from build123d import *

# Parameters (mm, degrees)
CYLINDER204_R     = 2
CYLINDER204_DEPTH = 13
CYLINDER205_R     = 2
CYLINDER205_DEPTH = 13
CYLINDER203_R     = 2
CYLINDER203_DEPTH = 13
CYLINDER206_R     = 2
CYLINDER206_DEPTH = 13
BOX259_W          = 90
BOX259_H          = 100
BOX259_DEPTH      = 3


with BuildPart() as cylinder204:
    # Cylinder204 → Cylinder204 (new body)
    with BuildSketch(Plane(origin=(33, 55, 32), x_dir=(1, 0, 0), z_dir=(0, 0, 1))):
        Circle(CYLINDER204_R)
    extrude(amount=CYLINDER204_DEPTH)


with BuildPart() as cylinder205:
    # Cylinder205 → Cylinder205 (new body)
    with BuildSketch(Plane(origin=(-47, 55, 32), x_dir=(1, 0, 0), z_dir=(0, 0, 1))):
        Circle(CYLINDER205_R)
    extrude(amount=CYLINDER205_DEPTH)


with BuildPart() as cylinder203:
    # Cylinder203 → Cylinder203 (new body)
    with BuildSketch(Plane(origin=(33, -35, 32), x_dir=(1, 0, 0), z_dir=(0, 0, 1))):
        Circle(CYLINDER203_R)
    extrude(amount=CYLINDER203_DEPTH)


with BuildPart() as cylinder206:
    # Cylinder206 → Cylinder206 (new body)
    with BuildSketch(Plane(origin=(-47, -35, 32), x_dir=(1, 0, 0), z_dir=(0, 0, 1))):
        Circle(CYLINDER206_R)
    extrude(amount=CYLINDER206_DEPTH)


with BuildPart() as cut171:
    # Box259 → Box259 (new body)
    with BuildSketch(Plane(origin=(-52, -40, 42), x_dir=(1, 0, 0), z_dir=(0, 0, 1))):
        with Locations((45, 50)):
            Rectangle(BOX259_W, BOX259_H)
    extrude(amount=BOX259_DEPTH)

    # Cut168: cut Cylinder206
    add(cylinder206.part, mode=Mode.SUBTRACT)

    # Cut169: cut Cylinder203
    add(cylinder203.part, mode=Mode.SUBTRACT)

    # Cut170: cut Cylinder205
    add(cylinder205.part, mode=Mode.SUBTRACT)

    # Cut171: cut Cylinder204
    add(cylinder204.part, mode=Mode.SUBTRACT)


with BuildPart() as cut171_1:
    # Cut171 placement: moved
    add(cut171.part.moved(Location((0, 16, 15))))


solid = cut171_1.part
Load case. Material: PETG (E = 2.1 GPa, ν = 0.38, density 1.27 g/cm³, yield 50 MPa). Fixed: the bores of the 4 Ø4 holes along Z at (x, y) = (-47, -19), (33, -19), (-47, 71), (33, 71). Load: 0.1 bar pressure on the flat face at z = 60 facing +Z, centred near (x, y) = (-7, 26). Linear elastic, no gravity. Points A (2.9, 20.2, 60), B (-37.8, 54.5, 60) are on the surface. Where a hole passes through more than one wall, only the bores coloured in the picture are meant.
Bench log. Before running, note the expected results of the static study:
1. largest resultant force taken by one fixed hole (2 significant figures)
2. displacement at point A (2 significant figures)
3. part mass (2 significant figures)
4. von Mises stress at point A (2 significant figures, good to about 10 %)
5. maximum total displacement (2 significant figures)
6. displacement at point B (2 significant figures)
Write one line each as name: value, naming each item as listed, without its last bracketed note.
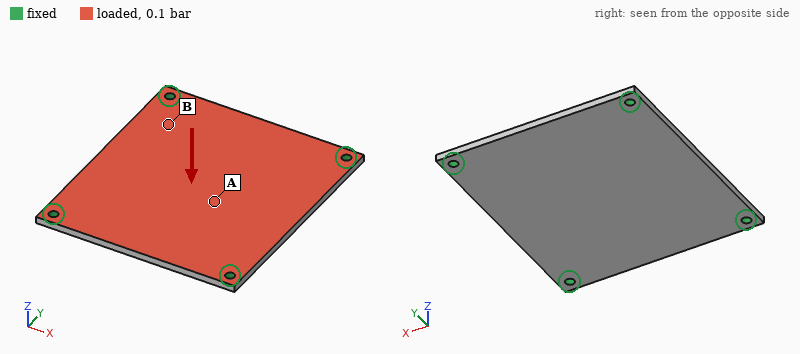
largest resultant force taken by one fixed hole: 22 N
displacement at point A: 0.77 mm
part mass: 34 g
von Mises stress at point A: 2.8 MPa
maximum total displacement: 0.80 mm
displacement at point B: 0.32 mm
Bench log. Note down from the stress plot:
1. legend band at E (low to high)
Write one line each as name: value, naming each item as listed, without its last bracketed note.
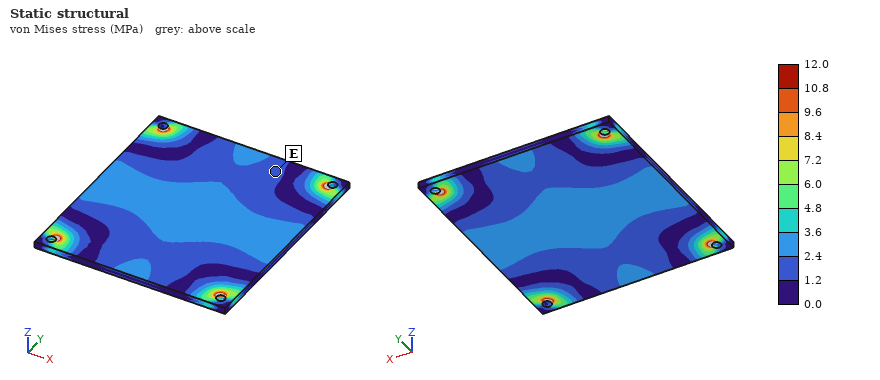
legend band at E: 1.2 to 2.4 MPa
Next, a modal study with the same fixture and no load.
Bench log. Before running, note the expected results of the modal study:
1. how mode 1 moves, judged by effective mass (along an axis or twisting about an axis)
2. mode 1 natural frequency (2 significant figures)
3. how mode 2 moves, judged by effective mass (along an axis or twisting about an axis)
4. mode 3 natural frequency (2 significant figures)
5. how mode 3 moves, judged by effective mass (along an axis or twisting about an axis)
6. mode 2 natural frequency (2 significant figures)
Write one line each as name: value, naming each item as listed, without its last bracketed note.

how mode 1 moves, judged by effective mass: along Z
mode 1 natural frequency: 340 Hz
how mode 2 moves, judged by effective mass: twisting about Y
mode 3 natural frequency: 650 Hz
how mode 3 moves, judged by effective mass: twisting about X
mode 2 natural frequency: 570 Hz
